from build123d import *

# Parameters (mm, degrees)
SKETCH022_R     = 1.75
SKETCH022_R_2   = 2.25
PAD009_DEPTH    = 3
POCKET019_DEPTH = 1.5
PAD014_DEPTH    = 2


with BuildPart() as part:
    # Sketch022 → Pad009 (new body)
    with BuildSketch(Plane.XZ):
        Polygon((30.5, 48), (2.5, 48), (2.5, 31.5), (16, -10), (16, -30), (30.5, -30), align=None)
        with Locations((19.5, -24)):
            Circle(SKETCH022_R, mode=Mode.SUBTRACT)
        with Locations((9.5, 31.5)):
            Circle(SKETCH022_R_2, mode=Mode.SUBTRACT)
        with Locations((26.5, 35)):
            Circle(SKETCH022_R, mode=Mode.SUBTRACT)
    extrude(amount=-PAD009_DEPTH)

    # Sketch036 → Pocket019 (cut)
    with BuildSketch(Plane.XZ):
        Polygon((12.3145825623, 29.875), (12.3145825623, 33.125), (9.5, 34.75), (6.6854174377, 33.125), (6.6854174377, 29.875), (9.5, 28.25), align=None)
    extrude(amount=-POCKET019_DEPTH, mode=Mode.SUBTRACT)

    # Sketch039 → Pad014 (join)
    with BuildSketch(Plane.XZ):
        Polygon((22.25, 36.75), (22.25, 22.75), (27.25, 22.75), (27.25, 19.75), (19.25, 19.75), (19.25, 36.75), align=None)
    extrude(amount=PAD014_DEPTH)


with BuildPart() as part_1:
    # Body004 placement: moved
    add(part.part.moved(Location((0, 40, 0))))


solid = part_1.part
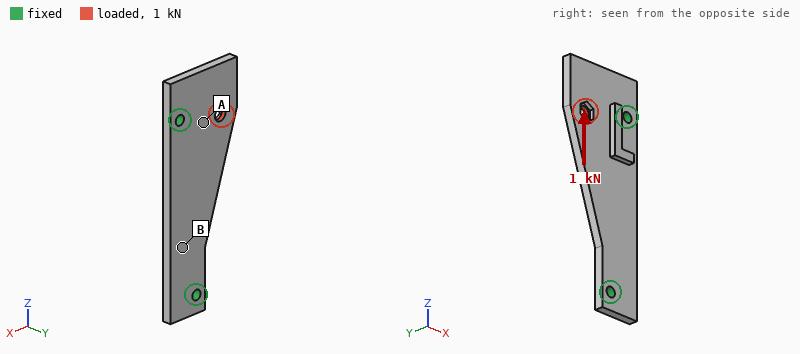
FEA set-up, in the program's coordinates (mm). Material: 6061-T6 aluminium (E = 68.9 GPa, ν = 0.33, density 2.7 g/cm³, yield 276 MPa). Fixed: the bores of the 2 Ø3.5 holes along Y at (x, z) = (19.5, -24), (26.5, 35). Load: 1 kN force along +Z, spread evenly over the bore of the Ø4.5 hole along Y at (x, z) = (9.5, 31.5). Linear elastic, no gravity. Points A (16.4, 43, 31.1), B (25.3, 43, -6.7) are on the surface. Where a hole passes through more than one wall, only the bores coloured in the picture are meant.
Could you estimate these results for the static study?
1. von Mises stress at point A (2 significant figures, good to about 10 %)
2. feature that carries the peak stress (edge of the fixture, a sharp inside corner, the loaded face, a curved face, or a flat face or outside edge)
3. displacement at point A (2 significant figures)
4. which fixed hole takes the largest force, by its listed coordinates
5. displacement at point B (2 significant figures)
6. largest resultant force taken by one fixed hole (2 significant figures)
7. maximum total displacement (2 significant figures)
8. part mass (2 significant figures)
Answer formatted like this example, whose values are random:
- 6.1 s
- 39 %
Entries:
- 23 MPa
- edge of the fixture
- 14 µm
- (26.5, 35)
- 16 µm
- 640 N
- 41 µm
- 13 g
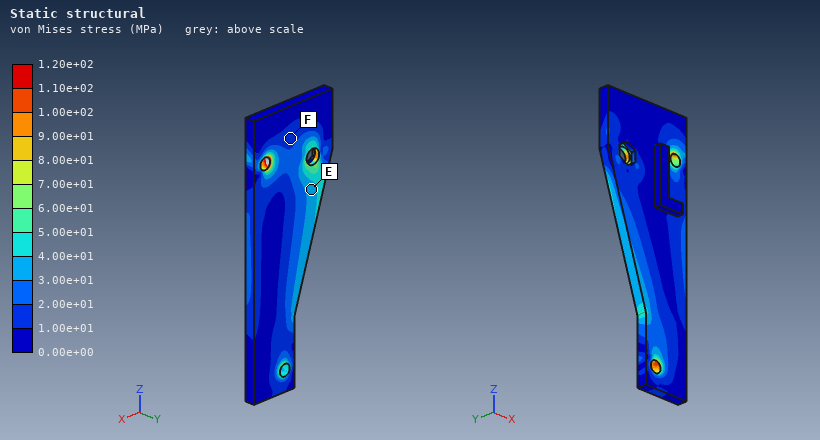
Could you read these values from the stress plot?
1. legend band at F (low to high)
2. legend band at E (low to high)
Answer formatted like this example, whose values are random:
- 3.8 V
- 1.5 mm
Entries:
- 1.00e+01 to 2.00e+01 MPa
- 3.00e+01 to 4.00e+01 MPa
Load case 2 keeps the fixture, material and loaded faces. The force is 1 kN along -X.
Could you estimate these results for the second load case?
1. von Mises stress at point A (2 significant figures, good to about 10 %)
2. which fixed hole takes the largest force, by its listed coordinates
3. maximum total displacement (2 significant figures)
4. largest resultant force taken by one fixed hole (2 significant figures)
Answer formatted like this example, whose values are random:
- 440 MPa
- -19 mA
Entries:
- 41 MPa
- (26.5, 35)
- 48 µm
- 950 N
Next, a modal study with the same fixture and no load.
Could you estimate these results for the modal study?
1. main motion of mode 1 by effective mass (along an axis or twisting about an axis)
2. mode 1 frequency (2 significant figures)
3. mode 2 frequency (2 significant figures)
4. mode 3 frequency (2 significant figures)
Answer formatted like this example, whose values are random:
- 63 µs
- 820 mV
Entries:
- along Y
- 3700 Hz
- 4400 Hz
- 7500 Hz
